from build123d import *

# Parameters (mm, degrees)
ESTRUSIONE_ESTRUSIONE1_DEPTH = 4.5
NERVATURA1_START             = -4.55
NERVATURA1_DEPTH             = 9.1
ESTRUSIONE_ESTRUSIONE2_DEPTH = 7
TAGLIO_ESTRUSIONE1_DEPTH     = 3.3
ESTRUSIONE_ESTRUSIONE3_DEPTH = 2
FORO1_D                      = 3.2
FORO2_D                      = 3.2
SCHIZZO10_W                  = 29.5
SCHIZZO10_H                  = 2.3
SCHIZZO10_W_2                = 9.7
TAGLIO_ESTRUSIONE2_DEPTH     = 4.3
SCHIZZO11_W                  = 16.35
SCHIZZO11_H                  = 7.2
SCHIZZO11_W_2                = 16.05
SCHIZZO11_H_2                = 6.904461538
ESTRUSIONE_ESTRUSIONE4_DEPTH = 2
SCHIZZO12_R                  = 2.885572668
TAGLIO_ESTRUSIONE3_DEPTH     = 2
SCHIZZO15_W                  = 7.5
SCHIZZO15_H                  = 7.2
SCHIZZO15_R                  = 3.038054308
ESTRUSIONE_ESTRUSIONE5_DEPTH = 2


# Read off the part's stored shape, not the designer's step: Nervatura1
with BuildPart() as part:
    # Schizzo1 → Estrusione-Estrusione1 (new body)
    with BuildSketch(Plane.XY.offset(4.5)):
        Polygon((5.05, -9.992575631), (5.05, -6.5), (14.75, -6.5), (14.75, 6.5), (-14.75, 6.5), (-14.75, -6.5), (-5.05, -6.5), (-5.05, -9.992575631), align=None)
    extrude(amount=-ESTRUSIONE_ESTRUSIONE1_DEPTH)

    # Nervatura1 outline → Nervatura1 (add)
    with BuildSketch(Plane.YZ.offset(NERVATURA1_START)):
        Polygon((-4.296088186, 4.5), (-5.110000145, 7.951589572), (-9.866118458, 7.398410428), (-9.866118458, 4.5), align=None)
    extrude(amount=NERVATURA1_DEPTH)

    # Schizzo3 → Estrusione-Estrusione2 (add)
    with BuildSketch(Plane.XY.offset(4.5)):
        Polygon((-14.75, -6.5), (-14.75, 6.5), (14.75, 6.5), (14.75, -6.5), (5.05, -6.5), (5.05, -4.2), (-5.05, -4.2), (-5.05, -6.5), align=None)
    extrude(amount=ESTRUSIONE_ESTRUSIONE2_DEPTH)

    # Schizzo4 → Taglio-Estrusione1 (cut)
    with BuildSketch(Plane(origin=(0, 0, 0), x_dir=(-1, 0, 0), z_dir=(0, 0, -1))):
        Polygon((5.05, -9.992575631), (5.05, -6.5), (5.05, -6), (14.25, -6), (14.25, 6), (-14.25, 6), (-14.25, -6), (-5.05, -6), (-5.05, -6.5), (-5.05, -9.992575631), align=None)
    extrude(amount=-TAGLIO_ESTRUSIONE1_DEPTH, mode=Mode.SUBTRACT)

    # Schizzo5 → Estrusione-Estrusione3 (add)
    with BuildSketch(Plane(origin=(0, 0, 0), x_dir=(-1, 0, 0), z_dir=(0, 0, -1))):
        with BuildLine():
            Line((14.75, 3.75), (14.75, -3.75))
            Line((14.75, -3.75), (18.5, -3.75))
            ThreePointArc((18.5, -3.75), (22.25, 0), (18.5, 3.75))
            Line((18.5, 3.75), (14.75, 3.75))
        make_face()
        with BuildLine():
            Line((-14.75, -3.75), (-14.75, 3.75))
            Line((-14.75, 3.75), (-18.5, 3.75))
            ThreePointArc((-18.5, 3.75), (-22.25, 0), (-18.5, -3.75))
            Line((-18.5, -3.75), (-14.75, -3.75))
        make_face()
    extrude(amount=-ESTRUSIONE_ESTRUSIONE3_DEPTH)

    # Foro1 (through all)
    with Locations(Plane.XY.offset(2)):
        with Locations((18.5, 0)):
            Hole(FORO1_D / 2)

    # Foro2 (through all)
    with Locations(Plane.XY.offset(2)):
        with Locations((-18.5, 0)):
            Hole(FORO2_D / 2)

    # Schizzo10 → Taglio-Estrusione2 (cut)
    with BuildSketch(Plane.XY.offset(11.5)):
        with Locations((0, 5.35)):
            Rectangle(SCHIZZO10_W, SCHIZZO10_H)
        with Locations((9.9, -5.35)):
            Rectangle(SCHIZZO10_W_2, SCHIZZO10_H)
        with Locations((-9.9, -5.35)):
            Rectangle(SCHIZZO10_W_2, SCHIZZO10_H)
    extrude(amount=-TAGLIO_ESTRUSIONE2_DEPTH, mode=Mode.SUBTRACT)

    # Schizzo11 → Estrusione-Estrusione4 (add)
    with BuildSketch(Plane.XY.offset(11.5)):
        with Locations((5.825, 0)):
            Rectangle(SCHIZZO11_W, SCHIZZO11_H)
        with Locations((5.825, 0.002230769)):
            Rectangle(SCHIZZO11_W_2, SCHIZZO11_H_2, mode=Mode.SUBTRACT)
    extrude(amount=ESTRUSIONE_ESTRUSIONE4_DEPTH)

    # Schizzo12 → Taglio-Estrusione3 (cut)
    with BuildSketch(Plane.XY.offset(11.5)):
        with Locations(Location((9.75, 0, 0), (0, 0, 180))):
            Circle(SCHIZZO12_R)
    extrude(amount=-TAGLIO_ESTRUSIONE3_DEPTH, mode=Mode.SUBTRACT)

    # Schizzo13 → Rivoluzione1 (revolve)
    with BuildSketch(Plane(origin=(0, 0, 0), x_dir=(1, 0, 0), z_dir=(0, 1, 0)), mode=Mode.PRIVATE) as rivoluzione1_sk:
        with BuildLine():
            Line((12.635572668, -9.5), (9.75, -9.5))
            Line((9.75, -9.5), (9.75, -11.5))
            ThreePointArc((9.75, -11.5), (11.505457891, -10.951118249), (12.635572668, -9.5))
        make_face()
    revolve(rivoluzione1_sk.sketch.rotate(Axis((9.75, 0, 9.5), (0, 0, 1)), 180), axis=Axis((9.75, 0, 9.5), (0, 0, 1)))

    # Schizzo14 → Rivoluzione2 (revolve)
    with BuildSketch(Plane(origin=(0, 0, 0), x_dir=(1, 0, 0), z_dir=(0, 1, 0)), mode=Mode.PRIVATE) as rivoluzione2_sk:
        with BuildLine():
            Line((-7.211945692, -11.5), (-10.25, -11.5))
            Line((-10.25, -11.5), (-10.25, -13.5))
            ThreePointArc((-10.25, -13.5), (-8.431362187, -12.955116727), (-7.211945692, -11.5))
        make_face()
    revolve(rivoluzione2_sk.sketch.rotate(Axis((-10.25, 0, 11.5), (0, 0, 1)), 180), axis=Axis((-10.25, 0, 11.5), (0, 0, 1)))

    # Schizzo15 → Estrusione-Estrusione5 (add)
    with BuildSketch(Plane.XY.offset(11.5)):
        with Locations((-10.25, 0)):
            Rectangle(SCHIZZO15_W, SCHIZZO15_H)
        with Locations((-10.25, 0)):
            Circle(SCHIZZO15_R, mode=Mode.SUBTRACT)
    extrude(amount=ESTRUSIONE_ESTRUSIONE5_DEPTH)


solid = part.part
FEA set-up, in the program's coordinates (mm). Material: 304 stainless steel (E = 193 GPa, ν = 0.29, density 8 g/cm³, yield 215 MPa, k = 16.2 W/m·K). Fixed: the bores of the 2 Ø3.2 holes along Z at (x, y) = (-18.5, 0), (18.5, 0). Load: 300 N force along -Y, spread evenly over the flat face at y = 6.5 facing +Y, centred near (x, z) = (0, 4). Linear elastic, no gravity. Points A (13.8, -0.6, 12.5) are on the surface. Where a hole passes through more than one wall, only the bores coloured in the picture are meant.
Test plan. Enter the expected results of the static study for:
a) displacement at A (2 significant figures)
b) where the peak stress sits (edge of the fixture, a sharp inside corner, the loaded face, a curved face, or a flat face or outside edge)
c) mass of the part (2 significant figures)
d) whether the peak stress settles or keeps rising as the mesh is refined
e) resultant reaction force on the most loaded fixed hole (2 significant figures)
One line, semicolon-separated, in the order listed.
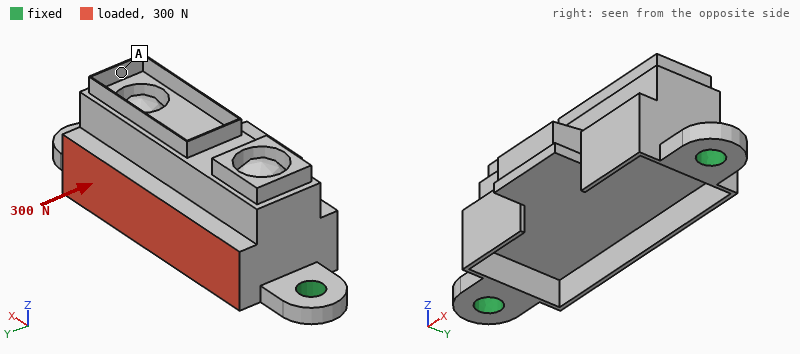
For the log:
10 µm; edge of the fixture; 24 g; keeps rising; 150 N
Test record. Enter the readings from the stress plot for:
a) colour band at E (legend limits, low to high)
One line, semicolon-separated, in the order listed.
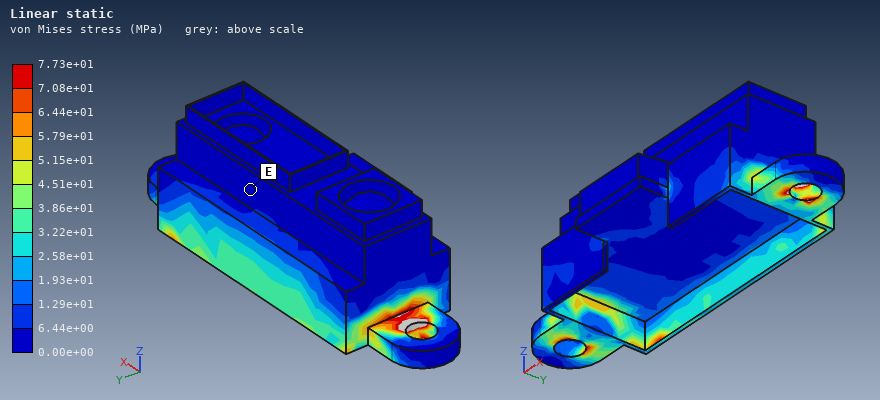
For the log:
0.00e+00 to 6.44e+00 MPa
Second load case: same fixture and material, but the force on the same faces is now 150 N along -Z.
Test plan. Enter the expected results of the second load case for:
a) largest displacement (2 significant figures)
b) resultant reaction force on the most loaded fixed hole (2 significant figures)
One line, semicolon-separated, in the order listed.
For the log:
14 µm; 83 N
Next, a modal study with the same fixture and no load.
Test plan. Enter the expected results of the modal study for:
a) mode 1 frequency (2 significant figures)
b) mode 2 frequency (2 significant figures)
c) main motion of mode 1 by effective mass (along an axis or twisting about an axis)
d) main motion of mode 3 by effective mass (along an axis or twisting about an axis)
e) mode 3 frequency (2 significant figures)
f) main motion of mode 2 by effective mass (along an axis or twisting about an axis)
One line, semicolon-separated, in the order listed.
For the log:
4300 Hz; 10 kHz; along Y; along Z; 12 kHz; along X
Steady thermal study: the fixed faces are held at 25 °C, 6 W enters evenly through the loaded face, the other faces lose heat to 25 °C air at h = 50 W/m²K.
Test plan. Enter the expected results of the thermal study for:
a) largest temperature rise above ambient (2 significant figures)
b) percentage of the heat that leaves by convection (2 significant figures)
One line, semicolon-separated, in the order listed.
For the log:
72 K; 68 %
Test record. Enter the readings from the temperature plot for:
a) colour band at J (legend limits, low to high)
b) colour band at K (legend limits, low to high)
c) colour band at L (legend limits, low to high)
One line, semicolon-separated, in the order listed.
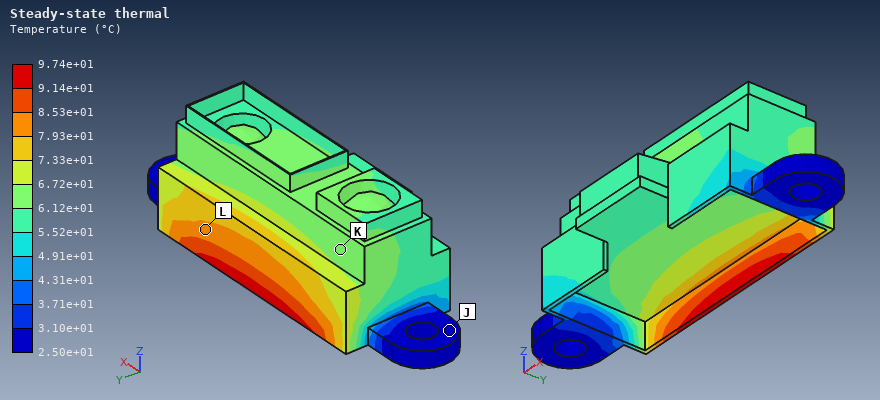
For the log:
2.50e+01 to 3.10e+01 °C; 6.12e+01 to 6.72e+01 °C; 7.93e+01 to 8.53e+01 °C
